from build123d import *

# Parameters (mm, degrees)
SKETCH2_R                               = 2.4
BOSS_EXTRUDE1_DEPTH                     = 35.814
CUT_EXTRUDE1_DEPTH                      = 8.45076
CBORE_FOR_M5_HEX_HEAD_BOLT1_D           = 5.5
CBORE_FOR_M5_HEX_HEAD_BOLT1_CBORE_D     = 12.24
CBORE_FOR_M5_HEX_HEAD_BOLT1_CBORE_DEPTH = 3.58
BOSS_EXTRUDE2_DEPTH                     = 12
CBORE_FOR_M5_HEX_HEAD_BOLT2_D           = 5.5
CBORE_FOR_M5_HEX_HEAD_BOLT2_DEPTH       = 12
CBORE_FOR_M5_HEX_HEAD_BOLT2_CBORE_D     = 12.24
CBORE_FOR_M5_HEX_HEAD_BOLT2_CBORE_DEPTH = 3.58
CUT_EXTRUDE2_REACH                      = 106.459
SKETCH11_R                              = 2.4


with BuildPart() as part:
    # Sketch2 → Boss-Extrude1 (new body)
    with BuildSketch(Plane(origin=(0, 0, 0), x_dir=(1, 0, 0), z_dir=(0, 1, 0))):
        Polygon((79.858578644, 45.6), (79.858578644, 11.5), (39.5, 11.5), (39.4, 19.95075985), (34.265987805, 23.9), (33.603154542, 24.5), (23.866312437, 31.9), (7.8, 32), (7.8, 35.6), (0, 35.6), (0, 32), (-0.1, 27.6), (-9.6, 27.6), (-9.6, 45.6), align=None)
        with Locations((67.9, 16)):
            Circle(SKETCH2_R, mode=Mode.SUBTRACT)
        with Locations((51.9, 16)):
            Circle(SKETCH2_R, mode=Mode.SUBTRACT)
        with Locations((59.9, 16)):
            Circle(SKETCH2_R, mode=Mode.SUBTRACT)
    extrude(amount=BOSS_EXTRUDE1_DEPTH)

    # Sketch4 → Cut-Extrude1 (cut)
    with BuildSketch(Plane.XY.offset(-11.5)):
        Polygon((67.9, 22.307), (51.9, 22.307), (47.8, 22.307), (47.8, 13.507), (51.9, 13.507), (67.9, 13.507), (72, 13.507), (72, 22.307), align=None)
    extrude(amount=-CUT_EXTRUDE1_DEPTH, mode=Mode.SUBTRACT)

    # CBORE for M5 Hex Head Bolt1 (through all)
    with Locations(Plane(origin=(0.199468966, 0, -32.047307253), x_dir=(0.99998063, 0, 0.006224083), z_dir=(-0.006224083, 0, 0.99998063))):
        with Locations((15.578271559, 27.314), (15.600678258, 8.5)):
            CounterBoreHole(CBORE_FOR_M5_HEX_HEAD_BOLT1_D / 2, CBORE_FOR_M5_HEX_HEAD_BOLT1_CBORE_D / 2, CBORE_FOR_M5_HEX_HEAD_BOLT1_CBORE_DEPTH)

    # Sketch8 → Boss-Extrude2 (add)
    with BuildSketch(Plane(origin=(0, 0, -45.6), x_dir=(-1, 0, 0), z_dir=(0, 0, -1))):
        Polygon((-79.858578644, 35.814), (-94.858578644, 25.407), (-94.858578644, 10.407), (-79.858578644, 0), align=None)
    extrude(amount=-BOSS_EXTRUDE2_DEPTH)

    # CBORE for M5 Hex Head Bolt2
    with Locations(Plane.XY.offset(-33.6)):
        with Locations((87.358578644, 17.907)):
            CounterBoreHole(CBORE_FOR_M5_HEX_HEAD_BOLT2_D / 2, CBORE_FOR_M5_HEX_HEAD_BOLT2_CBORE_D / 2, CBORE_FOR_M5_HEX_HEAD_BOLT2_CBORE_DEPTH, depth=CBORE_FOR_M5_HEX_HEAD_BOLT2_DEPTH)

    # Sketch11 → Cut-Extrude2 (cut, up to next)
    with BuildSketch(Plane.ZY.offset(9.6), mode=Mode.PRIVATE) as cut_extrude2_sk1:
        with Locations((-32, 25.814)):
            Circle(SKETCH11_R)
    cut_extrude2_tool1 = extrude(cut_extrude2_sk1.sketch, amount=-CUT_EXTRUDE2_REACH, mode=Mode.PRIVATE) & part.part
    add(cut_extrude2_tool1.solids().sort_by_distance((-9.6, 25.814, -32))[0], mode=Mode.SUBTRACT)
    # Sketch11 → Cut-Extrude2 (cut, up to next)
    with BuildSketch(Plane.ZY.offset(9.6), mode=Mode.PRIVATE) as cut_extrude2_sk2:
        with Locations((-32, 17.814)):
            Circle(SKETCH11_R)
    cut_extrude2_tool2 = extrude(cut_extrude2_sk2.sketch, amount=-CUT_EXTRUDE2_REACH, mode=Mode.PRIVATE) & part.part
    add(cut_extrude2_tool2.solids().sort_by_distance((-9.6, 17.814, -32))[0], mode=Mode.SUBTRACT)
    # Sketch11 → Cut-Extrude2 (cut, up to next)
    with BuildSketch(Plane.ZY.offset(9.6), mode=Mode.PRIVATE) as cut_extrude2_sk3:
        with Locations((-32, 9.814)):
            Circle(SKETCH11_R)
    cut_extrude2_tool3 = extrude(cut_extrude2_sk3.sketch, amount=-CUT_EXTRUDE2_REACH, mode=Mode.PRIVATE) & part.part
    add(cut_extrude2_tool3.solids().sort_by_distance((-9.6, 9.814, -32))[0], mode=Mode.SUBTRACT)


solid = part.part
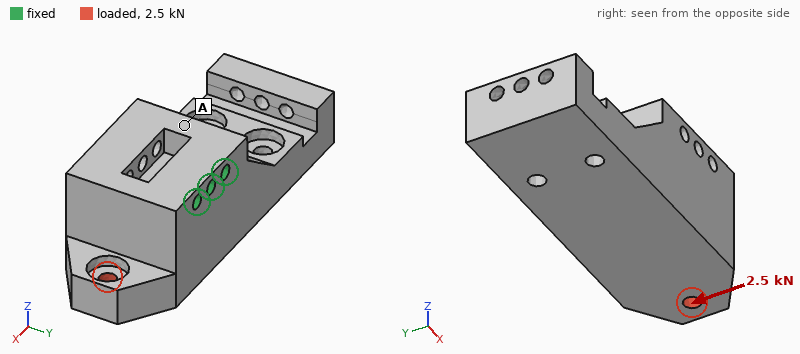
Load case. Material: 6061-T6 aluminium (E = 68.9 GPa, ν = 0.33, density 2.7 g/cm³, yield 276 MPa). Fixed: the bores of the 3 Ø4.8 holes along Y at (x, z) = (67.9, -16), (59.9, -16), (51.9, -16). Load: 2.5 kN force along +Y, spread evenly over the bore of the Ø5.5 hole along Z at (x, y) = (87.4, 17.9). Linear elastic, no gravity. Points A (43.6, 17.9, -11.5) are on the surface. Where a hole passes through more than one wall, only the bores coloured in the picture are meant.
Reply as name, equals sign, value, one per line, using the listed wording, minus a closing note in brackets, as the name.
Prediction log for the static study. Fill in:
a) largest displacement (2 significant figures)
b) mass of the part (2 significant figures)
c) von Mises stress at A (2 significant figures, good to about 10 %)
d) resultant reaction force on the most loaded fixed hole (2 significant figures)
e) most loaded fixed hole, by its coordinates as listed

largest displacement = 58 µm
mass of the part = 210 g
von Mises stress at A = 16 MPa
resultant reaction force on the most loaded fixed hole = 3.0 kN
most loaded fixed hole, by its coordinates as listed = (67.9, -16)
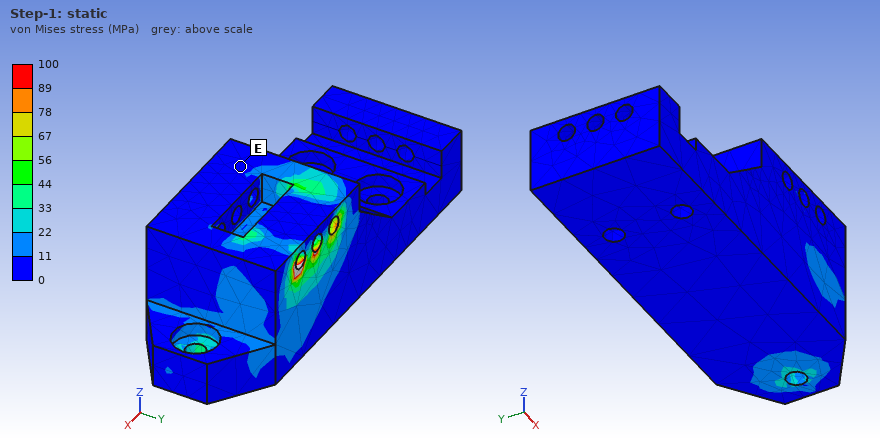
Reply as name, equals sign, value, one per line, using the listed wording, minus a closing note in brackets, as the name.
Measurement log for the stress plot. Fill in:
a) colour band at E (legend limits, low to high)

colour band at E = 0 to 11 MPa
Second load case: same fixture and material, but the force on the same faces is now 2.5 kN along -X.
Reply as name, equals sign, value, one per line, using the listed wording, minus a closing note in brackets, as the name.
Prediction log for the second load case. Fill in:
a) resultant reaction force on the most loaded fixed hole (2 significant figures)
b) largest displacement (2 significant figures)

resultant reaction force on the most loaded fixed hole = 3.2 kN
largest displacement = 29 µm
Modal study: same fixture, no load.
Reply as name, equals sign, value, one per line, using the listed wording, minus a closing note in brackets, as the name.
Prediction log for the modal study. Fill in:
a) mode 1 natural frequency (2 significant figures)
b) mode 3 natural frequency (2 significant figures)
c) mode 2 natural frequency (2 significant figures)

mode 1 natural frequency = 3000 Hz
mode 3 natural frequency = 4900 Hz
mode 2 natural frequency = 3500 Hz
